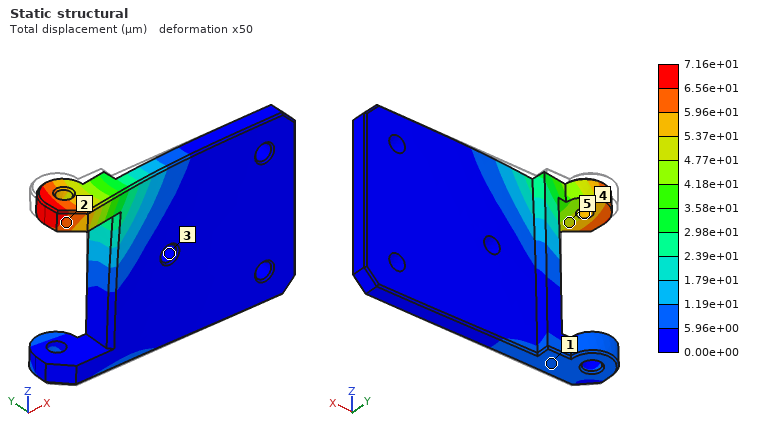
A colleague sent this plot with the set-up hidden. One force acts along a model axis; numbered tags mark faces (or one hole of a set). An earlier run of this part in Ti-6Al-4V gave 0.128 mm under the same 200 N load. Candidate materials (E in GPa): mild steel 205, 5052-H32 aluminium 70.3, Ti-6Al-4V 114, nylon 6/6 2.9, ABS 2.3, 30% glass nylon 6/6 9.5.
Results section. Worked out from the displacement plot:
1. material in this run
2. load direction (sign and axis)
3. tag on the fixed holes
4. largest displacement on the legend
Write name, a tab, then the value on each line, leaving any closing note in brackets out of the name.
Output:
material in this run	mild steel
load direction	-Y
tag on the fixed holes	3
largest displacement on the legend	7.16e+01 µm
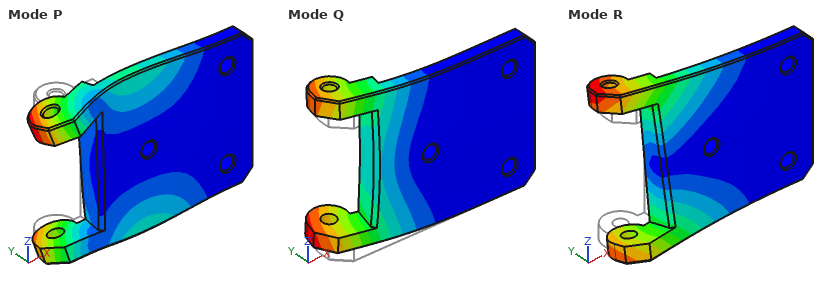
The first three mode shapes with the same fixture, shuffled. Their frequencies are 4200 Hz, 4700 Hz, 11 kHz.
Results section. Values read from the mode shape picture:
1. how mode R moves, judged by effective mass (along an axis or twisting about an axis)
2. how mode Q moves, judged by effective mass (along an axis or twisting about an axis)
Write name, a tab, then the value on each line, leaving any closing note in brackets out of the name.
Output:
how mode R moves, judged by effective mass	twisting about X
how mode Q moves, judged by effective mass	along Y
